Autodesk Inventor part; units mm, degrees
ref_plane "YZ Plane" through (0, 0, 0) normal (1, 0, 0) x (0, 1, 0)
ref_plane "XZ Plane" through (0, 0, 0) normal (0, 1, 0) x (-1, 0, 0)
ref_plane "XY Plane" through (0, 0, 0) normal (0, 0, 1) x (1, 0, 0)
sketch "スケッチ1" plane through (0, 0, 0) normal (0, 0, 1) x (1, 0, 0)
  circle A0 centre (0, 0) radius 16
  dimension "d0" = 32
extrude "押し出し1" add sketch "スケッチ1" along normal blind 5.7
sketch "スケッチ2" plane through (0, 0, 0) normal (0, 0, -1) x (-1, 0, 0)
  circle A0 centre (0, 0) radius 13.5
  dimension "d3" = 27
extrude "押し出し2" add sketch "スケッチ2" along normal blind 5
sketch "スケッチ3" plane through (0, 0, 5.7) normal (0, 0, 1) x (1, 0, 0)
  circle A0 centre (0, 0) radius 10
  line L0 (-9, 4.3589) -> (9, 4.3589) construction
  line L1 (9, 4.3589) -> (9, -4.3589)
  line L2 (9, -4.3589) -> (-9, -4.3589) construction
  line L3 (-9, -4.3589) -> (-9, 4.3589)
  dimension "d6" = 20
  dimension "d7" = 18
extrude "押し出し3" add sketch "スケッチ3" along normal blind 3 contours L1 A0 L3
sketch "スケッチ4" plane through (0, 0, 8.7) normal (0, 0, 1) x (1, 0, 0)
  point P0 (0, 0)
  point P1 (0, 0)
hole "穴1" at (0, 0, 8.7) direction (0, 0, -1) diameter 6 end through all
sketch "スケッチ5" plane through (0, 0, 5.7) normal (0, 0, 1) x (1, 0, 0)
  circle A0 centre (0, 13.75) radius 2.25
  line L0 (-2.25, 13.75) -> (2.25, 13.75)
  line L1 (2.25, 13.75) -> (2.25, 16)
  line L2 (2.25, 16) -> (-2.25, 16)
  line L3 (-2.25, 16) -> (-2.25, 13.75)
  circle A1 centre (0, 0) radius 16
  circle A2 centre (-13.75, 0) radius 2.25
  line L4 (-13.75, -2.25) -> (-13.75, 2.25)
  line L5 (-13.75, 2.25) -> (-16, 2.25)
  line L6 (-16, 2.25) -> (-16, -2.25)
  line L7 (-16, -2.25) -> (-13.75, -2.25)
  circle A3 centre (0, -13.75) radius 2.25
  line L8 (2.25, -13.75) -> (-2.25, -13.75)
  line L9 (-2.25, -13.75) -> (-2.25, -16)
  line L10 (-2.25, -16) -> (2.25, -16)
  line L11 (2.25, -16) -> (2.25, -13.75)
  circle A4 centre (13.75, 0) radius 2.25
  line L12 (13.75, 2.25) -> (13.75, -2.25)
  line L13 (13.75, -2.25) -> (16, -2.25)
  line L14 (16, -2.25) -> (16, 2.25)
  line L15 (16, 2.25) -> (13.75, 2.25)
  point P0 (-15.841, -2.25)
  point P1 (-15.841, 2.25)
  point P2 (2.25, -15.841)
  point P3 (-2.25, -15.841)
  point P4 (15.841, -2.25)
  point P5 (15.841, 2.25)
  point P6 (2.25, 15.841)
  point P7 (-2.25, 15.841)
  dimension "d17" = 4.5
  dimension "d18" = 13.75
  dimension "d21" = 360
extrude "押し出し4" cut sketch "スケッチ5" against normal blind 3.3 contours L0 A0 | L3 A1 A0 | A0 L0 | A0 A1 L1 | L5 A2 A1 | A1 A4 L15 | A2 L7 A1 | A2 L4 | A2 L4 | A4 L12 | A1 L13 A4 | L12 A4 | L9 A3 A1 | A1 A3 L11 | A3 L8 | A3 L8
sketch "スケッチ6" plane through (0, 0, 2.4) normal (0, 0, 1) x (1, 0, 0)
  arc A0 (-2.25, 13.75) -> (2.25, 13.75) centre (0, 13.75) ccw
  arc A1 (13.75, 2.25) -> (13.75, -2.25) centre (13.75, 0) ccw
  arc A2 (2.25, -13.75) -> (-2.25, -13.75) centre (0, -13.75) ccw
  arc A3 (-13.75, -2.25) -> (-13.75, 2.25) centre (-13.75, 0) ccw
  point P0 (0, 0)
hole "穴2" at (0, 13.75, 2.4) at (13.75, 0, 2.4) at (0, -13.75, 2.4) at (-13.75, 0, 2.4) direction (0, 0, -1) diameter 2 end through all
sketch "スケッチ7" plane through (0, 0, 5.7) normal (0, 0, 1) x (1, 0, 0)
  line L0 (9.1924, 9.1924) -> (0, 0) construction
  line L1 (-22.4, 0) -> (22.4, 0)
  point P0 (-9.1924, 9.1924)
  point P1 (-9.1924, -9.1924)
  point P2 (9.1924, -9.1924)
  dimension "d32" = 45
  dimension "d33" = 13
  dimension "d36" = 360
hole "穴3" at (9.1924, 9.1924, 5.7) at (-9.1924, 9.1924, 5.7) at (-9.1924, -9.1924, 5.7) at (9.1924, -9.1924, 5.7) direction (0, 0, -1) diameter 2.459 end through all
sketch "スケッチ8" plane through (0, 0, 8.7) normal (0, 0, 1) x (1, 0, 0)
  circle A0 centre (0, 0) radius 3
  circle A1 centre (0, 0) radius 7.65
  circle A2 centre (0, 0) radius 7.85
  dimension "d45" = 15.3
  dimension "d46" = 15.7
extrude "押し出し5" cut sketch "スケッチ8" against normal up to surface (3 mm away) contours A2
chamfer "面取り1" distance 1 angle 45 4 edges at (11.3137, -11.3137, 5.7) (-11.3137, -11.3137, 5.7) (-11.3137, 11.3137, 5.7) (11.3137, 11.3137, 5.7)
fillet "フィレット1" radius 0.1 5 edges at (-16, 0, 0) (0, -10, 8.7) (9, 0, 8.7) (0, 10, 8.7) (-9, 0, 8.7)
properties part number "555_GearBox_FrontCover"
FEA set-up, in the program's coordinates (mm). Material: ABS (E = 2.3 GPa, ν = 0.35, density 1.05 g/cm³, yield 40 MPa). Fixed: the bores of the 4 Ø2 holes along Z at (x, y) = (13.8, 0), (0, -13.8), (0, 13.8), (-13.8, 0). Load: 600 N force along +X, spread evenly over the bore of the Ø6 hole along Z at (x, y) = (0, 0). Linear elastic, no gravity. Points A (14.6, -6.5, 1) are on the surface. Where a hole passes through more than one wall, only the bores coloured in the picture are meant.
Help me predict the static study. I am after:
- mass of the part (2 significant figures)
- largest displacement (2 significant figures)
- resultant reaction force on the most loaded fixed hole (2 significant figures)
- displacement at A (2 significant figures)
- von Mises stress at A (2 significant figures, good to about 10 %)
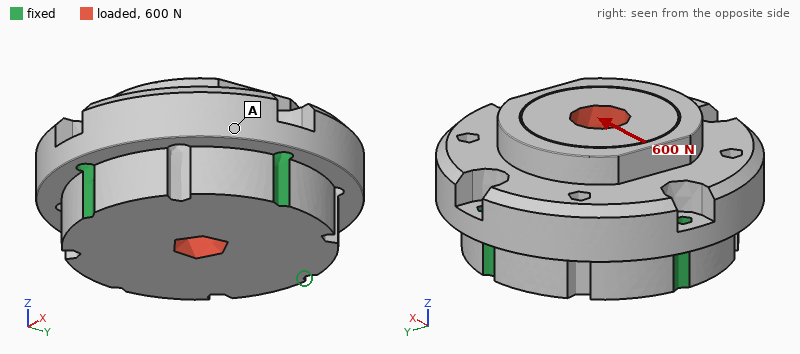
7.8 g
26 µm
200 N
12 µm
1.5 MPa
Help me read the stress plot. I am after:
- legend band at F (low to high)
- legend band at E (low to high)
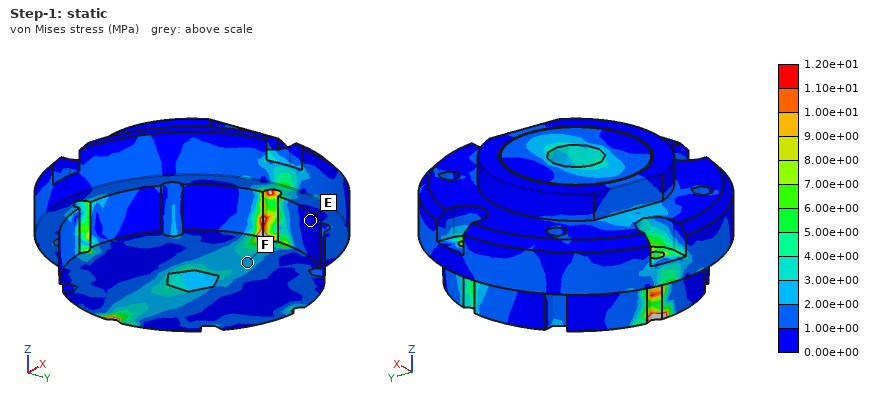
2.00e+00 to 3.00e+00 MPa
0.00e+00 to 1.00e+00 MPa
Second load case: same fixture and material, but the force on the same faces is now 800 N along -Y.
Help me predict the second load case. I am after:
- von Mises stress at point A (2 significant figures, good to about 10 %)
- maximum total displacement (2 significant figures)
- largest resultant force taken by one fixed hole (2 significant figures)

1.8 MPa
35 µm
270 N
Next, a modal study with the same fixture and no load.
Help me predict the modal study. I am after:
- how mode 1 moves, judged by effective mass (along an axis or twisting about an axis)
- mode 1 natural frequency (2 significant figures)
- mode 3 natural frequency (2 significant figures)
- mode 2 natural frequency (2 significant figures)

along Z
11 kHz
12 kHz
12 kHz
